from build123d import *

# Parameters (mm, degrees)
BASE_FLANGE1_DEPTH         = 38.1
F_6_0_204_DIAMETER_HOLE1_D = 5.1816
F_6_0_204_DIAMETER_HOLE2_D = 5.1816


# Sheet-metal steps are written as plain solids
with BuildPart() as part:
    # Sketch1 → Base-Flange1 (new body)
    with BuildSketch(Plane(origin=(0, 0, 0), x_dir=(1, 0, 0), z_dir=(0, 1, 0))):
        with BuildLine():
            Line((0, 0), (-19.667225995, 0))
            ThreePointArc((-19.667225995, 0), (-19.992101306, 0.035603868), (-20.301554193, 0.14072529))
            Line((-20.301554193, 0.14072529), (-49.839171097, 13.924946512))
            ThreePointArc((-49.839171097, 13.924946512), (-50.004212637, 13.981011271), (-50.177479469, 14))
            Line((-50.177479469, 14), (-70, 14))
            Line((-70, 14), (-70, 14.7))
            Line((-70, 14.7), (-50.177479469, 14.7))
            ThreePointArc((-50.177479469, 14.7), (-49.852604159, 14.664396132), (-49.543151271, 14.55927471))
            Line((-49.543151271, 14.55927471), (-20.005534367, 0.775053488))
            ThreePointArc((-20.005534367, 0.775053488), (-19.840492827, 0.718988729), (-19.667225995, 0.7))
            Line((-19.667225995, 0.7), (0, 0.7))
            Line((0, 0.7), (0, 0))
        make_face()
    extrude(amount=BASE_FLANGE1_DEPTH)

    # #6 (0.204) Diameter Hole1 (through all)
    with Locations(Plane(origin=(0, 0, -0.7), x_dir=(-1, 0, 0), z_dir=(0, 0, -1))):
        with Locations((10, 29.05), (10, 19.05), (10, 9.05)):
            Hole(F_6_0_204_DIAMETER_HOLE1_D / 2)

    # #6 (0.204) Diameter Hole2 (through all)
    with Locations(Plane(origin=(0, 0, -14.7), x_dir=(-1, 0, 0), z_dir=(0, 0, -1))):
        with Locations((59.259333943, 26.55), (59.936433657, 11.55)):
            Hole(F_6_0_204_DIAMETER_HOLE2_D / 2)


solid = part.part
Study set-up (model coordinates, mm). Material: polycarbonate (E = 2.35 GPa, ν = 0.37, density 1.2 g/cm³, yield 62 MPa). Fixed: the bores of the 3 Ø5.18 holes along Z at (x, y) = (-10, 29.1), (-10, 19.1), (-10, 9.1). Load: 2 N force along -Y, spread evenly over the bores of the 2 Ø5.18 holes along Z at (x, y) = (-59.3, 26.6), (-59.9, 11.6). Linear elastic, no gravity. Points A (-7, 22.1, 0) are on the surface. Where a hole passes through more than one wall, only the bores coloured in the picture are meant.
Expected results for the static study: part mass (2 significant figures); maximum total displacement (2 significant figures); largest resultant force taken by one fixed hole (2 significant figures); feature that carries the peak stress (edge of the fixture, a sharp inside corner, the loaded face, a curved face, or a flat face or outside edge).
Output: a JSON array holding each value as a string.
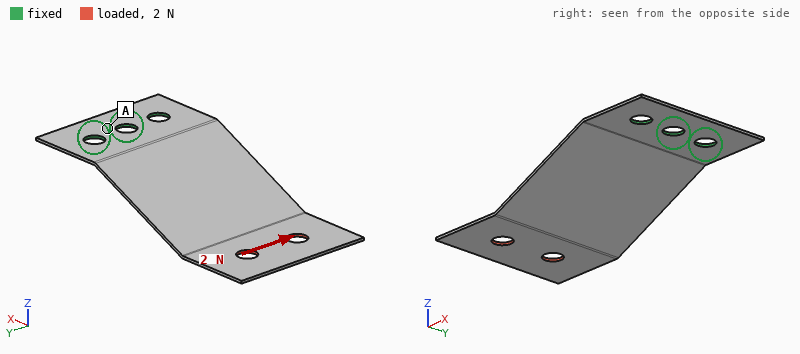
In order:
["2.3 g", "0.92 mm", "4.4 N", "a flat face or outside edge"]
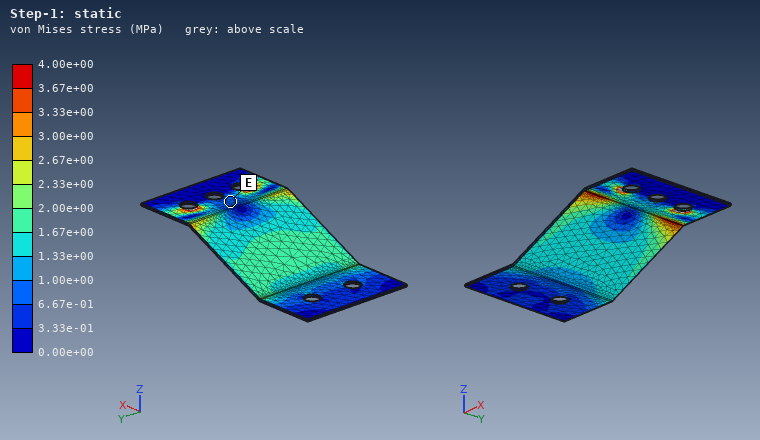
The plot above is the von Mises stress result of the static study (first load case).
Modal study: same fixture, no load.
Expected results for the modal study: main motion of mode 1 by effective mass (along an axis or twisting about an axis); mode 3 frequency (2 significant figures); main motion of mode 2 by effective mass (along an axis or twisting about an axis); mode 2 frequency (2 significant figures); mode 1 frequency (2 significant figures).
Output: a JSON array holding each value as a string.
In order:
["along Z", "280 Hz", "twisting about X", "150 Hz", "46 Hz"]
